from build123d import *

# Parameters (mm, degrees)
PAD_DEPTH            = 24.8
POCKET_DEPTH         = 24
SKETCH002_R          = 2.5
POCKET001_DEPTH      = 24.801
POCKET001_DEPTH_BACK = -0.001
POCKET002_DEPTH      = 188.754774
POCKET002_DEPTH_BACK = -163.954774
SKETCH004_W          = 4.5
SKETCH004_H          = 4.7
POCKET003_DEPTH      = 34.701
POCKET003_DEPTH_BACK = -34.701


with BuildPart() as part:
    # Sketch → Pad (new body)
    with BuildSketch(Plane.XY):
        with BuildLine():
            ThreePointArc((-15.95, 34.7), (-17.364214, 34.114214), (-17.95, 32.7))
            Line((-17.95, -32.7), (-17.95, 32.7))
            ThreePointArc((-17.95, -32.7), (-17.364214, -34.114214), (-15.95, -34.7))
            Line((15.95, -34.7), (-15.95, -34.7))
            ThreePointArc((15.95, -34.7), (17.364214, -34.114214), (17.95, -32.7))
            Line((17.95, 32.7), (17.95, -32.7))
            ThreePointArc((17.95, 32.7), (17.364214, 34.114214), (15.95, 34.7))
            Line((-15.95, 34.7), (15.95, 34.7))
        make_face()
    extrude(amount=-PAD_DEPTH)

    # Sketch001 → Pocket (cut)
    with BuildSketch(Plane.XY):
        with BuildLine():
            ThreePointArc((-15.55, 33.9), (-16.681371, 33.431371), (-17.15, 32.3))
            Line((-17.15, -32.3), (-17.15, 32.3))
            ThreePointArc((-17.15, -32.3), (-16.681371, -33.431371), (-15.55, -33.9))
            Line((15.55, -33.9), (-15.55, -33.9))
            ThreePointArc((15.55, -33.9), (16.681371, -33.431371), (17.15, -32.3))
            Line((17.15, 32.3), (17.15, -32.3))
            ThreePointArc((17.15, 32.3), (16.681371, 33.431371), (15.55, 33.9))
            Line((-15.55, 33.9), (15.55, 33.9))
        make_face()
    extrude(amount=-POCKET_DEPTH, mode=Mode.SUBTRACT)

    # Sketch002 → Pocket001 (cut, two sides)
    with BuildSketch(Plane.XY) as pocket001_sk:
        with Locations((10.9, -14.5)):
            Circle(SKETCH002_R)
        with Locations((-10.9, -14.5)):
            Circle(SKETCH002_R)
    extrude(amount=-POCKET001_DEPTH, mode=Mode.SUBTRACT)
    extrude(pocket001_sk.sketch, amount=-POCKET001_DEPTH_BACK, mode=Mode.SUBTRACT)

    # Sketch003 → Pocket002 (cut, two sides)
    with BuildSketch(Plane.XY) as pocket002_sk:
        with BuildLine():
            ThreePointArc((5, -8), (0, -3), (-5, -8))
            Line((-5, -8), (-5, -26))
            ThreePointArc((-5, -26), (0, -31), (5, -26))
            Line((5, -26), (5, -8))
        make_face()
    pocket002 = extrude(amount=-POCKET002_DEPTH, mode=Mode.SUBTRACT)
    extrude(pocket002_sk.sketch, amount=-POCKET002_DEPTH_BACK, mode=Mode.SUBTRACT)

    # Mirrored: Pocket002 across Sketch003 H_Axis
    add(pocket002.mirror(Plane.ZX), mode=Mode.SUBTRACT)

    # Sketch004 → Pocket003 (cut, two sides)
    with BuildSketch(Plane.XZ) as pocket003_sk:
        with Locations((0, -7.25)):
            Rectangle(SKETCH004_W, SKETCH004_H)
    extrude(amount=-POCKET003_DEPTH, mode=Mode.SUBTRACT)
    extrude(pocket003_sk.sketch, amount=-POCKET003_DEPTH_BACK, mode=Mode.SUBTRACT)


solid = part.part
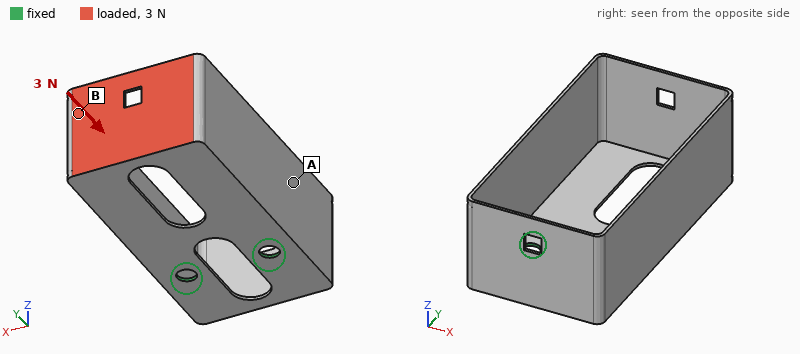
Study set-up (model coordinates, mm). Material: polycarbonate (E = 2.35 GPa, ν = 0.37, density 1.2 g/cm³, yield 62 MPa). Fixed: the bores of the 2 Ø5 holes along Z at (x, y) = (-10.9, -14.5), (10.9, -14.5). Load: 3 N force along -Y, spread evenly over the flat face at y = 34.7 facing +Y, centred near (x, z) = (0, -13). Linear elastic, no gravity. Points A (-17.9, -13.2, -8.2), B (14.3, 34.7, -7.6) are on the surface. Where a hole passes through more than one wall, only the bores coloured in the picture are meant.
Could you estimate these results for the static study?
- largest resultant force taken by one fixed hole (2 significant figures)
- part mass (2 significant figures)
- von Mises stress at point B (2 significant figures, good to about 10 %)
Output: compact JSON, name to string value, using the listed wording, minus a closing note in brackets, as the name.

{"largest resultant force taken by one fixed hole": "1.5 N", "part mass": "6.6 g", "von Mises stress at point B": "1.1 MPa"}
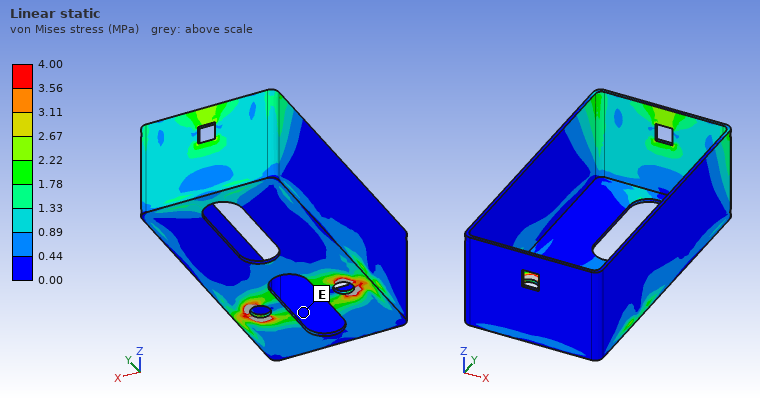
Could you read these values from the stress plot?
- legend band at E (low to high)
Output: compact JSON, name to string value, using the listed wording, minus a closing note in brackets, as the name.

{"legend band at E": "0.00 to 0.44 MPa"}
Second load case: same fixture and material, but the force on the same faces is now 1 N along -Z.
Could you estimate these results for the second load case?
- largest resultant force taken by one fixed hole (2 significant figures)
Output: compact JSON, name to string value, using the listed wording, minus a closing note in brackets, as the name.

{"largest resultant force taken by one fixed hole": "0.50 N"}
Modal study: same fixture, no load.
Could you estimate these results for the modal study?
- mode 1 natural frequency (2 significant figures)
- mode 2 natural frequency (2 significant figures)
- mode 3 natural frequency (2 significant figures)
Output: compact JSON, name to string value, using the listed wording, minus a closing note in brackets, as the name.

{"mode 1 natural frequency": "110 Hz", "mode 2 natural frequency": "160 Hz", "mode 3 natural frequency": "360 Hz"}
